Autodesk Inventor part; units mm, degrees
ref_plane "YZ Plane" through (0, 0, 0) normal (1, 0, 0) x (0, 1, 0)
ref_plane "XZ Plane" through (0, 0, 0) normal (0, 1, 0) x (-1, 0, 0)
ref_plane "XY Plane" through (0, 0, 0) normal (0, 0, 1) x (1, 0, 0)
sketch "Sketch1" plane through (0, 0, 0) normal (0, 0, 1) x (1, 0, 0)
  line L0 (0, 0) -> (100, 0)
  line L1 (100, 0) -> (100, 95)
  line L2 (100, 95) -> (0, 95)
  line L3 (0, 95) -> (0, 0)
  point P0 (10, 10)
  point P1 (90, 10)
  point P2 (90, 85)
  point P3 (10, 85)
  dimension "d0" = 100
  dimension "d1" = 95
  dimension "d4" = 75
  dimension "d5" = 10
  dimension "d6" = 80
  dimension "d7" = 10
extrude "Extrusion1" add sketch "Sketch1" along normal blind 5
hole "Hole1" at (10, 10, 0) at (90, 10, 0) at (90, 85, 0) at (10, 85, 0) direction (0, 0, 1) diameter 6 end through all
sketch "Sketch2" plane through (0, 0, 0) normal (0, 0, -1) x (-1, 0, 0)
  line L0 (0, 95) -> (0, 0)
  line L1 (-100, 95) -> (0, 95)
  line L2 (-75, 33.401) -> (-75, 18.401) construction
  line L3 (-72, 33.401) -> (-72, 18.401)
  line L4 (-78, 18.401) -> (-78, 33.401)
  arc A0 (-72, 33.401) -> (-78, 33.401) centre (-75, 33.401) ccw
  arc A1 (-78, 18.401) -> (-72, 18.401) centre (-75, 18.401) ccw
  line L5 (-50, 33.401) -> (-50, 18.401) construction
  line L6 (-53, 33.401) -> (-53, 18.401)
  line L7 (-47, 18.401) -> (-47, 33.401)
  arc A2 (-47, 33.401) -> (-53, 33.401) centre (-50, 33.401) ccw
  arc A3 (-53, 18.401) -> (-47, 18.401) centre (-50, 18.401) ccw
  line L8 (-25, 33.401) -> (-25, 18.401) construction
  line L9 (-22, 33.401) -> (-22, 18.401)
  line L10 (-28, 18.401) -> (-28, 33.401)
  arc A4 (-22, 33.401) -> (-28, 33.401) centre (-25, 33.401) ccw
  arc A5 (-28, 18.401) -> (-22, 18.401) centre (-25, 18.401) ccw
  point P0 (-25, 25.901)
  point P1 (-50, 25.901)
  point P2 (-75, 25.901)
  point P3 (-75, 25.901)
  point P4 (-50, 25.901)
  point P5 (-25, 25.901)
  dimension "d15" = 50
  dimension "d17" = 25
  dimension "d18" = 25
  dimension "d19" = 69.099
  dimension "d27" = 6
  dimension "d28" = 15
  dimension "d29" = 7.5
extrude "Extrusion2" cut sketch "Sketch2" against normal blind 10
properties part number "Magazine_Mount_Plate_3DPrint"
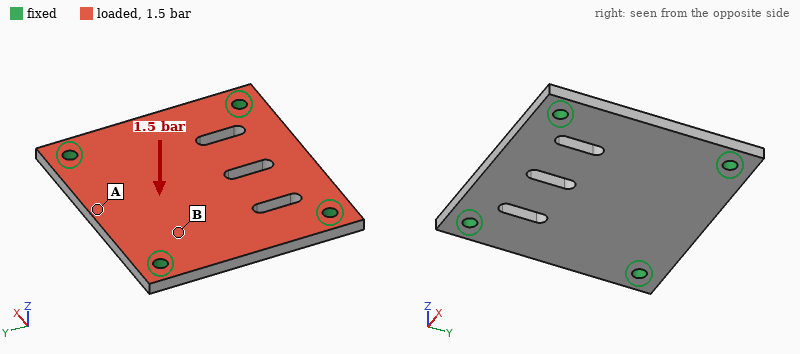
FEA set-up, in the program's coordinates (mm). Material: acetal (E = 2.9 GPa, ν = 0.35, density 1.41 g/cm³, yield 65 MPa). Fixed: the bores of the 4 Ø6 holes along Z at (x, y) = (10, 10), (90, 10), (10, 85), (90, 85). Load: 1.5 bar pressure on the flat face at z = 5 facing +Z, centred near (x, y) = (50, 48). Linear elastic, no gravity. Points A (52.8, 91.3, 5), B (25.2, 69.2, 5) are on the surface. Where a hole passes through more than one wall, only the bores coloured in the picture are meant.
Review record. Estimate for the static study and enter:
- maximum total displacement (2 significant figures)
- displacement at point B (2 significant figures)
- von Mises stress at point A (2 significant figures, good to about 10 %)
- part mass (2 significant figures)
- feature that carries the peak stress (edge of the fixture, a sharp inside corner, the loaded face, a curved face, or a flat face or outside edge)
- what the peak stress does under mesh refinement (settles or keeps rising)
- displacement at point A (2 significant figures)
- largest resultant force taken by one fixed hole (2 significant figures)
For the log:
1.2 mm
0.57 mm
11 MPa
64 g
edge of the fixture
keeps rising
0.59 mm
350 N
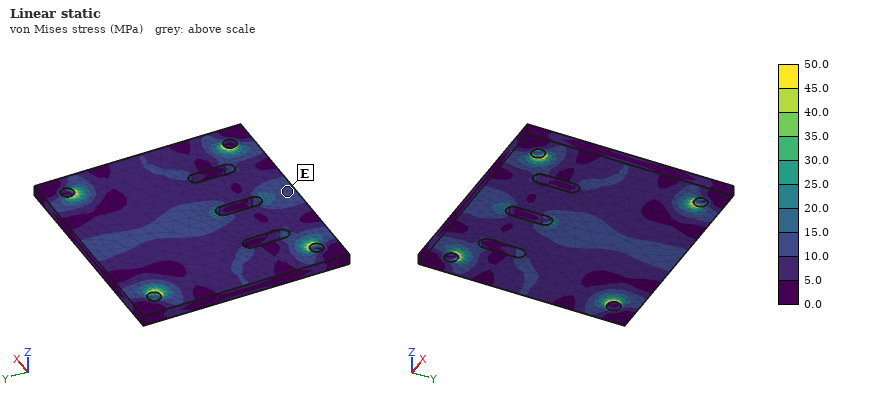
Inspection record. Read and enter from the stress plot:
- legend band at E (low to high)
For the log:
10.0 to 15.0 MPa
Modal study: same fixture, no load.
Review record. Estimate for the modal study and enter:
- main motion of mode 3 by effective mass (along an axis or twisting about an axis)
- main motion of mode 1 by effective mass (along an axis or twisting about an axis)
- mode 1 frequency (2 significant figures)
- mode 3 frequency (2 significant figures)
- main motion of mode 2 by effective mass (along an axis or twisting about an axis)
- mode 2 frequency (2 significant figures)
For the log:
twisting about Y
along Z
830 Hz
1400 Hz
twisting about X
1300 Hz
